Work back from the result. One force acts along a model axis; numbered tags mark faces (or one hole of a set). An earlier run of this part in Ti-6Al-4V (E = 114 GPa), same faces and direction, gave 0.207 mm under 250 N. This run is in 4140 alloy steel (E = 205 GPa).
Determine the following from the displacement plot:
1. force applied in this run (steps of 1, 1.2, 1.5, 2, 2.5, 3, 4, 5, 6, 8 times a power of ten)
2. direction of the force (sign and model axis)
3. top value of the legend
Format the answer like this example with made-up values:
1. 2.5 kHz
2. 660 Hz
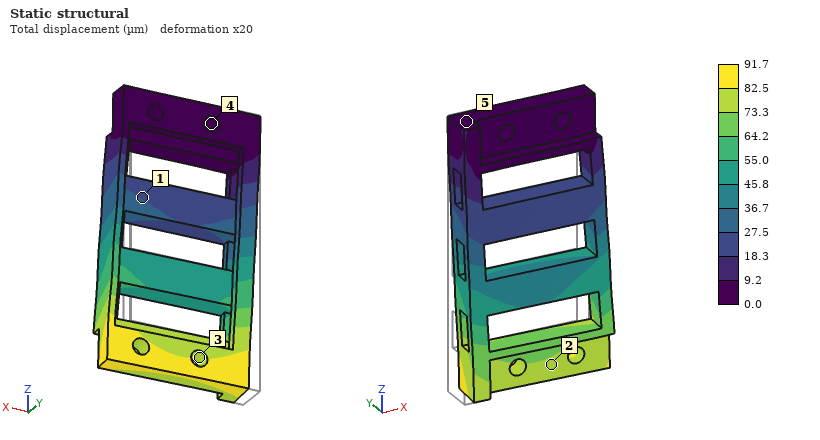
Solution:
1. 200 N
2. +X
3. 91.7 µm
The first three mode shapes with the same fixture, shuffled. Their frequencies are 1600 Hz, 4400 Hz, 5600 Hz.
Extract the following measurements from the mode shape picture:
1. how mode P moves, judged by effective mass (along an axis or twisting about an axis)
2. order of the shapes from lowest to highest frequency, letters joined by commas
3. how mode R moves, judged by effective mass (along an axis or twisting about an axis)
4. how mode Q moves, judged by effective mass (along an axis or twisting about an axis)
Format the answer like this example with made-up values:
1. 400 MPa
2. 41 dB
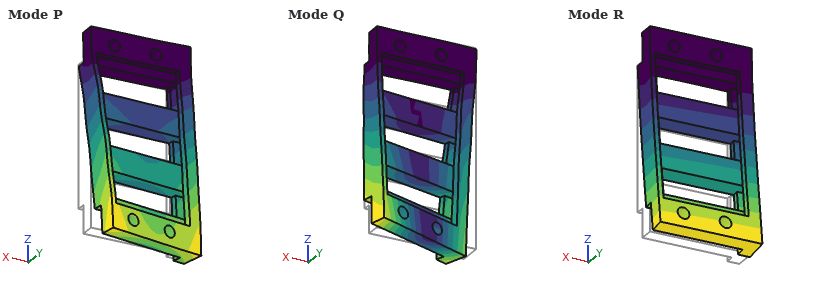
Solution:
1. along X
2. R, P, Q
3. along Y
4. along X
